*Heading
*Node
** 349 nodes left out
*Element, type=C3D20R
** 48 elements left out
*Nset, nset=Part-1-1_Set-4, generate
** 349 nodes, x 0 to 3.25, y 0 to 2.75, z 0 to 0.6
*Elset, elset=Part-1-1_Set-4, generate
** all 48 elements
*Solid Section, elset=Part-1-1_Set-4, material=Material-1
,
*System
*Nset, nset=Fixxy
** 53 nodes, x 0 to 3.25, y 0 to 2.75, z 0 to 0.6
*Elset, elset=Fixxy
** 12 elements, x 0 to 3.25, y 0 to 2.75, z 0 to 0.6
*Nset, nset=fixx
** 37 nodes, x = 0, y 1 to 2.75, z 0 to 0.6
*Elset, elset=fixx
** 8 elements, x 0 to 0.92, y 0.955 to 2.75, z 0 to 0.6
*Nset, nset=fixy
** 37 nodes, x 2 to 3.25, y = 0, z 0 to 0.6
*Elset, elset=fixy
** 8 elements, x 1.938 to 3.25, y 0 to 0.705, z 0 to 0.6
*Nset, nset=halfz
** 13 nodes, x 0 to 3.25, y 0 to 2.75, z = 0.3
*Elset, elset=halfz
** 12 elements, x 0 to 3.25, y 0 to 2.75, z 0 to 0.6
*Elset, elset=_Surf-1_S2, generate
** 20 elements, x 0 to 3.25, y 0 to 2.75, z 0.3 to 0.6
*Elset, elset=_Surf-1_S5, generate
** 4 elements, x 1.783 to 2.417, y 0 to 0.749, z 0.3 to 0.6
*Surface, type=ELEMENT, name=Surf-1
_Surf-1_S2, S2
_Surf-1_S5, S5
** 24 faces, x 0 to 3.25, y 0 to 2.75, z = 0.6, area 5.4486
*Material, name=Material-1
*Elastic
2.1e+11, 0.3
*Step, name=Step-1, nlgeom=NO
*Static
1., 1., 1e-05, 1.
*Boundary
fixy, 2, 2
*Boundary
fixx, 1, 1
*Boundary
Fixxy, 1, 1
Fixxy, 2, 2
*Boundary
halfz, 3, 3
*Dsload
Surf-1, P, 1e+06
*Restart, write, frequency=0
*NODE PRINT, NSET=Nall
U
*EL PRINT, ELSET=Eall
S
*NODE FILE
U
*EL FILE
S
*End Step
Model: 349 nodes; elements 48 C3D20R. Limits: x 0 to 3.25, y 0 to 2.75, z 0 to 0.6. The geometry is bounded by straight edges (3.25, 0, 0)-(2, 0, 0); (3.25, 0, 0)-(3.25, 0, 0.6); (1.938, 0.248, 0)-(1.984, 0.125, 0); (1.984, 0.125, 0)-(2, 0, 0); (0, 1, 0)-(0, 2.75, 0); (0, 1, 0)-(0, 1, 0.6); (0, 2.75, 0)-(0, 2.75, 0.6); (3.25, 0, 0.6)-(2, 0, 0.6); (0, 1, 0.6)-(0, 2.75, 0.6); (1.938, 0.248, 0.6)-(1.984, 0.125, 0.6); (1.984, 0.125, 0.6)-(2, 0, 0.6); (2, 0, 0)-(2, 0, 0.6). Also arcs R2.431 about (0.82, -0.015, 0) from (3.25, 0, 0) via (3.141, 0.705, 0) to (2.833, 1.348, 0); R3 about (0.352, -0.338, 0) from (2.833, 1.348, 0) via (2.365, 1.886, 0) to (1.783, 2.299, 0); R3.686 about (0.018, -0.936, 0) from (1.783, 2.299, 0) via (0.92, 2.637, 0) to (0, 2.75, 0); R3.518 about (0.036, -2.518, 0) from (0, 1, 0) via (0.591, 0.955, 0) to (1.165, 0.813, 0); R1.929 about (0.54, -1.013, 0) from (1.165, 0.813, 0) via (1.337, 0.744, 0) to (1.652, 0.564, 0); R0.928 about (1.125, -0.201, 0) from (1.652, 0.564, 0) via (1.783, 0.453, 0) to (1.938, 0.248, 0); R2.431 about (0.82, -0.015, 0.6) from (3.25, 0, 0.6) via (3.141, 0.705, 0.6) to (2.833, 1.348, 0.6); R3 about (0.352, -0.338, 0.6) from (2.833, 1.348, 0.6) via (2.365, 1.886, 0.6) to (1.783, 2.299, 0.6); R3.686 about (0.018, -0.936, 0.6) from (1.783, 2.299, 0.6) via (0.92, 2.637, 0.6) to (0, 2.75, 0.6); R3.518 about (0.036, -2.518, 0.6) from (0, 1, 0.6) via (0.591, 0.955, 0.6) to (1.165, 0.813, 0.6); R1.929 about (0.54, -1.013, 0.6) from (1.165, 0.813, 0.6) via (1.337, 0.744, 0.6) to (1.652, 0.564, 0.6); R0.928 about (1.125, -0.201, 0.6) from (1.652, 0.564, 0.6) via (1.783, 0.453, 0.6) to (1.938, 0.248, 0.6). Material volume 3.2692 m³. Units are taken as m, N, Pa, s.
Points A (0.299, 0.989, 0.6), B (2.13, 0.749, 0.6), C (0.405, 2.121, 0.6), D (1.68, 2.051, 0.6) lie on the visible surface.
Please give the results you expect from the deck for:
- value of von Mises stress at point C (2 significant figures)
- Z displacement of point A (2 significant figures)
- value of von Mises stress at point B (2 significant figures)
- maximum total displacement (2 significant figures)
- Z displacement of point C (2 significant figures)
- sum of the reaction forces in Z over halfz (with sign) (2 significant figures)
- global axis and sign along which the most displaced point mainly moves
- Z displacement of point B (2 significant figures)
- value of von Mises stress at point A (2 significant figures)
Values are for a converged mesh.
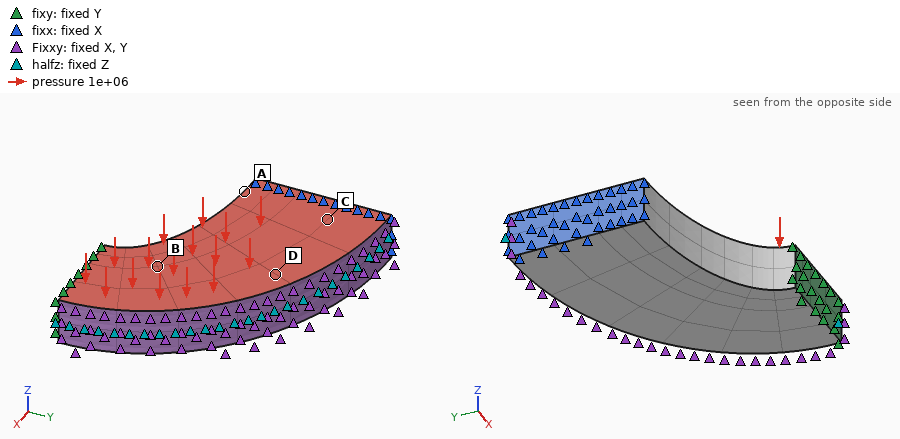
6.0e+06 Pa
-2.0e-04 m
4.1e+06 Pa
2.0e-04 m
-5.5e-05 m
5.4e+06 N
-Z
-7.4e-05 m
4.7e+06 Pa
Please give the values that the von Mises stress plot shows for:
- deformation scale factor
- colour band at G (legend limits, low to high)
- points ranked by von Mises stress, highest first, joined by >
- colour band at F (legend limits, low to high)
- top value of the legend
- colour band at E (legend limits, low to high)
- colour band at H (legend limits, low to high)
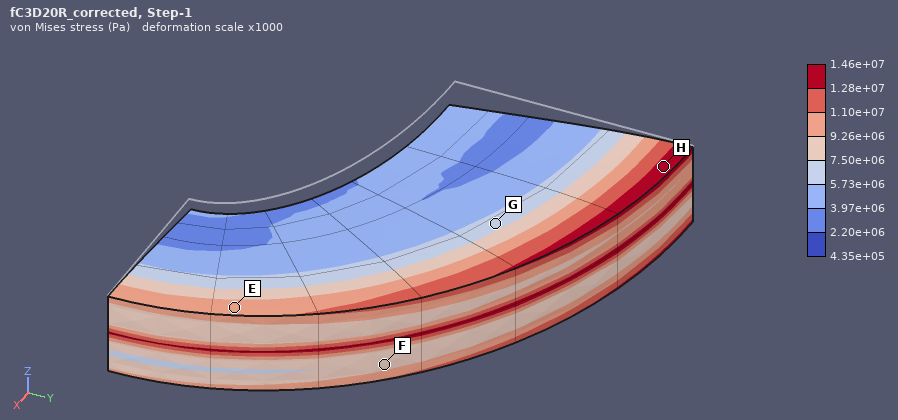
1000
5.73e+06 to 7.50e+06 Pa
H > E > F > G
7.50e+06 to 9.26e+06 Pa
1.46e+07 Pa
9.26e+06 to 1.10e+07 Pa
1.28e+07 to 1.46e+07 Pa
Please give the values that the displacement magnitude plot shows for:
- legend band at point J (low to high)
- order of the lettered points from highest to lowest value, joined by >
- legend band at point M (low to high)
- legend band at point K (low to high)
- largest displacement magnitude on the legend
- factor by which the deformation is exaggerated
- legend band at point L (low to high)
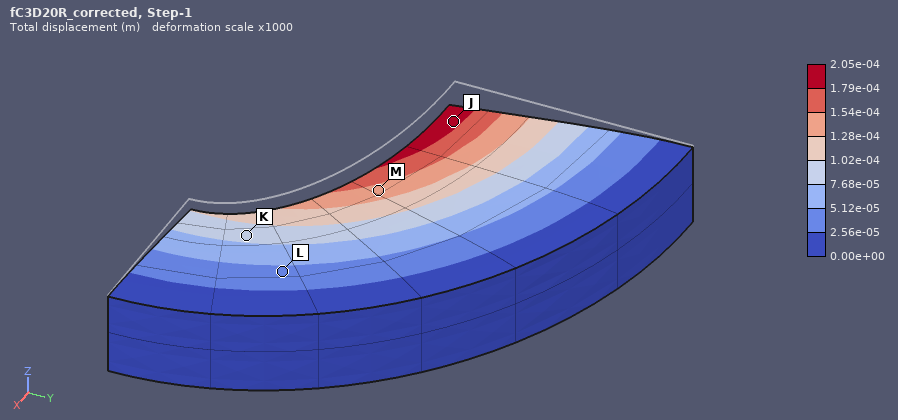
1.79e-04 to 2.05e-04 m
J > M > K > L
1.28e-04 to 1.54e-04 m
7.68e-05 to 1.02e-04 m
2.05e-04 m
1000
2.56e-05 to 5.12e-05 m
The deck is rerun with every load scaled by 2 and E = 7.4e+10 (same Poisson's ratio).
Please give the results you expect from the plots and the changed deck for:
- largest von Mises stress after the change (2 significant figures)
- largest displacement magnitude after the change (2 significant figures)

2.9e+07 Pa
0.0012 m
